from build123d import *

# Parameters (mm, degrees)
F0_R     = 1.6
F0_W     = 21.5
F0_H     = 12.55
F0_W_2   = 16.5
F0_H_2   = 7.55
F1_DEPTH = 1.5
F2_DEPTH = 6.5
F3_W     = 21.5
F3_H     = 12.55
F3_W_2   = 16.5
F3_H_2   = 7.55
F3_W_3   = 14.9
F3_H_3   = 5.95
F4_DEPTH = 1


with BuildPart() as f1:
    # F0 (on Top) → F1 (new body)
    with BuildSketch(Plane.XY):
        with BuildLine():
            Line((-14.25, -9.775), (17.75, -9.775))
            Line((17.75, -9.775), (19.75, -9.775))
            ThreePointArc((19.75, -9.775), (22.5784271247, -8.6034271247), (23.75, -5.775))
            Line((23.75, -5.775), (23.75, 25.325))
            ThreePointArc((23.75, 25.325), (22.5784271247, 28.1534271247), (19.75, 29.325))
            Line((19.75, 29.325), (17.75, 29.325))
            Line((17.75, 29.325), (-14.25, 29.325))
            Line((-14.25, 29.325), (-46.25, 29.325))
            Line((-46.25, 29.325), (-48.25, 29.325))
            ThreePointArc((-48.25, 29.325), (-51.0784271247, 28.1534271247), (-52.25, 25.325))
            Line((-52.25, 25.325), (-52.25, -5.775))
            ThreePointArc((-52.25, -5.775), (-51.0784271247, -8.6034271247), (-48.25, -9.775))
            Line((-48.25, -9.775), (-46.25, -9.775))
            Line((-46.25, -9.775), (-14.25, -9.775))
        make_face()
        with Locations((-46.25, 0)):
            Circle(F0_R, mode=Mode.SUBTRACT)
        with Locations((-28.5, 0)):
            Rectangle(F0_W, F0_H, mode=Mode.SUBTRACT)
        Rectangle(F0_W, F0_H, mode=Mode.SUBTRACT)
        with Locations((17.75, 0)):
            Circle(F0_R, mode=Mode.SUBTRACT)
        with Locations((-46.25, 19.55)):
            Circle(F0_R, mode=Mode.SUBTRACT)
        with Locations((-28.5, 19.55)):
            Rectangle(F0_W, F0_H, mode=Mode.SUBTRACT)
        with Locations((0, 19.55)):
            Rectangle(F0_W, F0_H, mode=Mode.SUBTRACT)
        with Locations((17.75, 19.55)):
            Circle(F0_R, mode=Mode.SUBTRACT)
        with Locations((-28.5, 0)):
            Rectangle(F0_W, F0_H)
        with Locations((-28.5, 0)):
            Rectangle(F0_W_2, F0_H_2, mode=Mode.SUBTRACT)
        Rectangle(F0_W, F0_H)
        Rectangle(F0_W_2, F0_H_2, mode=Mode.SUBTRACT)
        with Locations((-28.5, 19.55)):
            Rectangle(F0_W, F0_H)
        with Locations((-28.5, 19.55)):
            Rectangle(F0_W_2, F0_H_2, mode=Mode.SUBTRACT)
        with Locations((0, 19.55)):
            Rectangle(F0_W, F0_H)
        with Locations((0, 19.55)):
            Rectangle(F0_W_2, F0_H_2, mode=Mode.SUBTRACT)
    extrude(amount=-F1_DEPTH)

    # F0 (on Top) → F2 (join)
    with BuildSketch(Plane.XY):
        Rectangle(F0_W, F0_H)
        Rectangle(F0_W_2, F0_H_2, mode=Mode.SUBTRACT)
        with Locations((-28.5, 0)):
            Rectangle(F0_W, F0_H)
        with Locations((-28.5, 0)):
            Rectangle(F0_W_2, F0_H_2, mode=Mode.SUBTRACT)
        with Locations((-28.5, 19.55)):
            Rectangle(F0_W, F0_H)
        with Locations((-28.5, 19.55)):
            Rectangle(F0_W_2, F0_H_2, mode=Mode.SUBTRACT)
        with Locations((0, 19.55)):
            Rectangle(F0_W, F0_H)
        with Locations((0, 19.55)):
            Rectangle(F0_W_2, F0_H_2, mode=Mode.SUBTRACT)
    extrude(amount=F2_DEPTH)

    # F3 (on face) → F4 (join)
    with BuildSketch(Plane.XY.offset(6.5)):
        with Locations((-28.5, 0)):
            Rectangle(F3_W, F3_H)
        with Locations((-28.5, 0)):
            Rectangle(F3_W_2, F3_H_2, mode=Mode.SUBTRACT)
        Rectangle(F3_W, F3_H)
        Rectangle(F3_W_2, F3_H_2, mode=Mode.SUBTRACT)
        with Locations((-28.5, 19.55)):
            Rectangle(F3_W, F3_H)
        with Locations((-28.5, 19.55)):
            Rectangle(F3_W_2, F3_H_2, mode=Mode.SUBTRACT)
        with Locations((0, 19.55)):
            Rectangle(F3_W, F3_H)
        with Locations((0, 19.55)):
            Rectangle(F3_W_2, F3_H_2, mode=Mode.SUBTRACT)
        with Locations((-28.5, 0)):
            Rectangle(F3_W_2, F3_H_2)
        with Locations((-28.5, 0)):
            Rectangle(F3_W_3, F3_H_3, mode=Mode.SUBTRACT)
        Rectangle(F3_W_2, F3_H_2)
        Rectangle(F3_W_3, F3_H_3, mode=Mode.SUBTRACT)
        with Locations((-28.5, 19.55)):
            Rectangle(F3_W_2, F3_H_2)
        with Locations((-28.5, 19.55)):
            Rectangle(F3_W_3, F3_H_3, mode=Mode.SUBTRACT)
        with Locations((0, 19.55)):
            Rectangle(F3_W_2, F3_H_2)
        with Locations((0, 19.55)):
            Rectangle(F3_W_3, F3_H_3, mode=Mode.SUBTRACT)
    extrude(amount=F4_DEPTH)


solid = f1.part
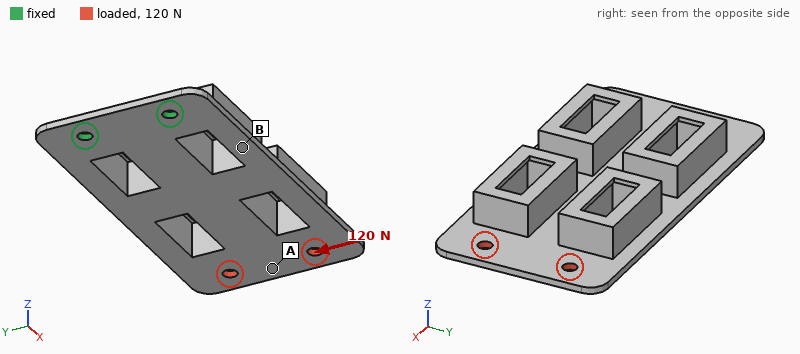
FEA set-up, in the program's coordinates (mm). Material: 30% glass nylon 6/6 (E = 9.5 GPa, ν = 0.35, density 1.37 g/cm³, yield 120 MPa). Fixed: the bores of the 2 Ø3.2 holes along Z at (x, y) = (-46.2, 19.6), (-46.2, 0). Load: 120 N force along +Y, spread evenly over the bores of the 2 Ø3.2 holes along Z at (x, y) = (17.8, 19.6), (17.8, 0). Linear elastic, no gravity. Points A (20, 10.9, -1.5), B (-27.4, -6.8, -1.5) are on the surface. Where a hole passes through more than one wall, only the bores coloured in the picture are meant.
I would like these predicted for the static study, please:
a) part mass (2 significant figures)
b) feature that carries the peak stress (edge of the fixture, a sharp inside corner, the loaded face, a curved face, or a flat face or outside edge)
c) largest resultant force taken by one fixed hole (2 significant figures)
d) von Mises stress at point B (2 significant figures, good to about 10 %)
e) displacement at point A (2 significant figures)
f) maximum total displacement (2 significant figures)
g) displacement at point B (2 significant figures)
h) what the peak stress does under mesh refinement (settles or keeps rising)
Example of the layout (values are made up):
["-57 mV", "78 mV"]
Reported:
["11 g", "edge of the fixture", "360 N", "14 MPa", "0.38 mm", "0.44 mm", "0.12 mm", "keeps rising"]
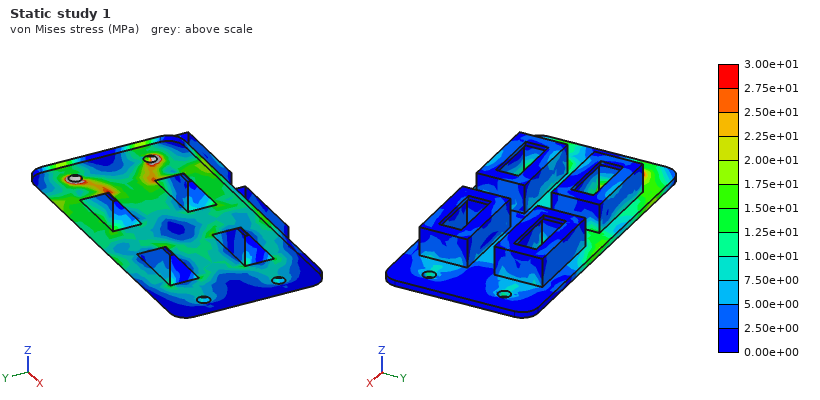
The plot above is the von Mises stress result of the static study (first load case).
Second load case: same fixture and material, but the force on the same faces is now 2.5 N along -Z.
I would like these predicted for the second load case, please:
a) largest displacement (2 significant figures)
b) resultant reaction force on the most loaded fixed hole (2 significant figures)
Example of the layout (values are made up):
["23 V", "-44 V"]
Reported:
["0.98 mm", "1.3 N"]
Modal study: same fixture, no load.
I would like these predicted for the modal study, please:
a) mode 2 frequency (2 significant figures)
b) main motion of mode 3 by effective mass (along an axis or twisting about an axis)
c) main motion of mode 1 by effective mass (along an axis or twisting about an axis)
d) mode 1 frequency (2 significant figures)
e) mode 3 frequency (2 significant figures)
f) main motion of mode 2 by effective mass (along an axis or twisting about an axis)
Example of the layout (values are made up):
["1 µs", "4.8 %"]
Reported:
["810 Hz", "along Z", "along Z", "150 Hz", "920 Hz", "twisting about X"]
